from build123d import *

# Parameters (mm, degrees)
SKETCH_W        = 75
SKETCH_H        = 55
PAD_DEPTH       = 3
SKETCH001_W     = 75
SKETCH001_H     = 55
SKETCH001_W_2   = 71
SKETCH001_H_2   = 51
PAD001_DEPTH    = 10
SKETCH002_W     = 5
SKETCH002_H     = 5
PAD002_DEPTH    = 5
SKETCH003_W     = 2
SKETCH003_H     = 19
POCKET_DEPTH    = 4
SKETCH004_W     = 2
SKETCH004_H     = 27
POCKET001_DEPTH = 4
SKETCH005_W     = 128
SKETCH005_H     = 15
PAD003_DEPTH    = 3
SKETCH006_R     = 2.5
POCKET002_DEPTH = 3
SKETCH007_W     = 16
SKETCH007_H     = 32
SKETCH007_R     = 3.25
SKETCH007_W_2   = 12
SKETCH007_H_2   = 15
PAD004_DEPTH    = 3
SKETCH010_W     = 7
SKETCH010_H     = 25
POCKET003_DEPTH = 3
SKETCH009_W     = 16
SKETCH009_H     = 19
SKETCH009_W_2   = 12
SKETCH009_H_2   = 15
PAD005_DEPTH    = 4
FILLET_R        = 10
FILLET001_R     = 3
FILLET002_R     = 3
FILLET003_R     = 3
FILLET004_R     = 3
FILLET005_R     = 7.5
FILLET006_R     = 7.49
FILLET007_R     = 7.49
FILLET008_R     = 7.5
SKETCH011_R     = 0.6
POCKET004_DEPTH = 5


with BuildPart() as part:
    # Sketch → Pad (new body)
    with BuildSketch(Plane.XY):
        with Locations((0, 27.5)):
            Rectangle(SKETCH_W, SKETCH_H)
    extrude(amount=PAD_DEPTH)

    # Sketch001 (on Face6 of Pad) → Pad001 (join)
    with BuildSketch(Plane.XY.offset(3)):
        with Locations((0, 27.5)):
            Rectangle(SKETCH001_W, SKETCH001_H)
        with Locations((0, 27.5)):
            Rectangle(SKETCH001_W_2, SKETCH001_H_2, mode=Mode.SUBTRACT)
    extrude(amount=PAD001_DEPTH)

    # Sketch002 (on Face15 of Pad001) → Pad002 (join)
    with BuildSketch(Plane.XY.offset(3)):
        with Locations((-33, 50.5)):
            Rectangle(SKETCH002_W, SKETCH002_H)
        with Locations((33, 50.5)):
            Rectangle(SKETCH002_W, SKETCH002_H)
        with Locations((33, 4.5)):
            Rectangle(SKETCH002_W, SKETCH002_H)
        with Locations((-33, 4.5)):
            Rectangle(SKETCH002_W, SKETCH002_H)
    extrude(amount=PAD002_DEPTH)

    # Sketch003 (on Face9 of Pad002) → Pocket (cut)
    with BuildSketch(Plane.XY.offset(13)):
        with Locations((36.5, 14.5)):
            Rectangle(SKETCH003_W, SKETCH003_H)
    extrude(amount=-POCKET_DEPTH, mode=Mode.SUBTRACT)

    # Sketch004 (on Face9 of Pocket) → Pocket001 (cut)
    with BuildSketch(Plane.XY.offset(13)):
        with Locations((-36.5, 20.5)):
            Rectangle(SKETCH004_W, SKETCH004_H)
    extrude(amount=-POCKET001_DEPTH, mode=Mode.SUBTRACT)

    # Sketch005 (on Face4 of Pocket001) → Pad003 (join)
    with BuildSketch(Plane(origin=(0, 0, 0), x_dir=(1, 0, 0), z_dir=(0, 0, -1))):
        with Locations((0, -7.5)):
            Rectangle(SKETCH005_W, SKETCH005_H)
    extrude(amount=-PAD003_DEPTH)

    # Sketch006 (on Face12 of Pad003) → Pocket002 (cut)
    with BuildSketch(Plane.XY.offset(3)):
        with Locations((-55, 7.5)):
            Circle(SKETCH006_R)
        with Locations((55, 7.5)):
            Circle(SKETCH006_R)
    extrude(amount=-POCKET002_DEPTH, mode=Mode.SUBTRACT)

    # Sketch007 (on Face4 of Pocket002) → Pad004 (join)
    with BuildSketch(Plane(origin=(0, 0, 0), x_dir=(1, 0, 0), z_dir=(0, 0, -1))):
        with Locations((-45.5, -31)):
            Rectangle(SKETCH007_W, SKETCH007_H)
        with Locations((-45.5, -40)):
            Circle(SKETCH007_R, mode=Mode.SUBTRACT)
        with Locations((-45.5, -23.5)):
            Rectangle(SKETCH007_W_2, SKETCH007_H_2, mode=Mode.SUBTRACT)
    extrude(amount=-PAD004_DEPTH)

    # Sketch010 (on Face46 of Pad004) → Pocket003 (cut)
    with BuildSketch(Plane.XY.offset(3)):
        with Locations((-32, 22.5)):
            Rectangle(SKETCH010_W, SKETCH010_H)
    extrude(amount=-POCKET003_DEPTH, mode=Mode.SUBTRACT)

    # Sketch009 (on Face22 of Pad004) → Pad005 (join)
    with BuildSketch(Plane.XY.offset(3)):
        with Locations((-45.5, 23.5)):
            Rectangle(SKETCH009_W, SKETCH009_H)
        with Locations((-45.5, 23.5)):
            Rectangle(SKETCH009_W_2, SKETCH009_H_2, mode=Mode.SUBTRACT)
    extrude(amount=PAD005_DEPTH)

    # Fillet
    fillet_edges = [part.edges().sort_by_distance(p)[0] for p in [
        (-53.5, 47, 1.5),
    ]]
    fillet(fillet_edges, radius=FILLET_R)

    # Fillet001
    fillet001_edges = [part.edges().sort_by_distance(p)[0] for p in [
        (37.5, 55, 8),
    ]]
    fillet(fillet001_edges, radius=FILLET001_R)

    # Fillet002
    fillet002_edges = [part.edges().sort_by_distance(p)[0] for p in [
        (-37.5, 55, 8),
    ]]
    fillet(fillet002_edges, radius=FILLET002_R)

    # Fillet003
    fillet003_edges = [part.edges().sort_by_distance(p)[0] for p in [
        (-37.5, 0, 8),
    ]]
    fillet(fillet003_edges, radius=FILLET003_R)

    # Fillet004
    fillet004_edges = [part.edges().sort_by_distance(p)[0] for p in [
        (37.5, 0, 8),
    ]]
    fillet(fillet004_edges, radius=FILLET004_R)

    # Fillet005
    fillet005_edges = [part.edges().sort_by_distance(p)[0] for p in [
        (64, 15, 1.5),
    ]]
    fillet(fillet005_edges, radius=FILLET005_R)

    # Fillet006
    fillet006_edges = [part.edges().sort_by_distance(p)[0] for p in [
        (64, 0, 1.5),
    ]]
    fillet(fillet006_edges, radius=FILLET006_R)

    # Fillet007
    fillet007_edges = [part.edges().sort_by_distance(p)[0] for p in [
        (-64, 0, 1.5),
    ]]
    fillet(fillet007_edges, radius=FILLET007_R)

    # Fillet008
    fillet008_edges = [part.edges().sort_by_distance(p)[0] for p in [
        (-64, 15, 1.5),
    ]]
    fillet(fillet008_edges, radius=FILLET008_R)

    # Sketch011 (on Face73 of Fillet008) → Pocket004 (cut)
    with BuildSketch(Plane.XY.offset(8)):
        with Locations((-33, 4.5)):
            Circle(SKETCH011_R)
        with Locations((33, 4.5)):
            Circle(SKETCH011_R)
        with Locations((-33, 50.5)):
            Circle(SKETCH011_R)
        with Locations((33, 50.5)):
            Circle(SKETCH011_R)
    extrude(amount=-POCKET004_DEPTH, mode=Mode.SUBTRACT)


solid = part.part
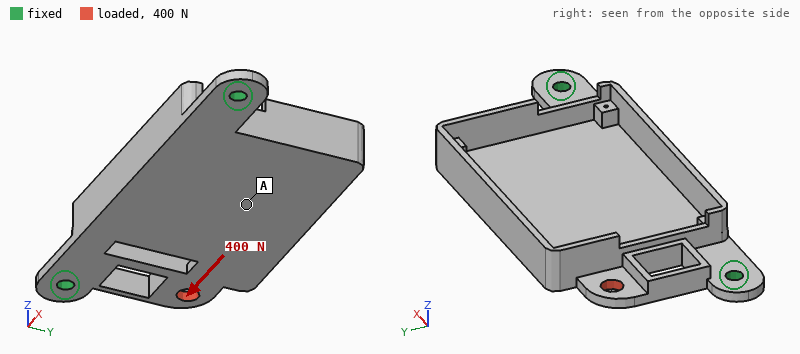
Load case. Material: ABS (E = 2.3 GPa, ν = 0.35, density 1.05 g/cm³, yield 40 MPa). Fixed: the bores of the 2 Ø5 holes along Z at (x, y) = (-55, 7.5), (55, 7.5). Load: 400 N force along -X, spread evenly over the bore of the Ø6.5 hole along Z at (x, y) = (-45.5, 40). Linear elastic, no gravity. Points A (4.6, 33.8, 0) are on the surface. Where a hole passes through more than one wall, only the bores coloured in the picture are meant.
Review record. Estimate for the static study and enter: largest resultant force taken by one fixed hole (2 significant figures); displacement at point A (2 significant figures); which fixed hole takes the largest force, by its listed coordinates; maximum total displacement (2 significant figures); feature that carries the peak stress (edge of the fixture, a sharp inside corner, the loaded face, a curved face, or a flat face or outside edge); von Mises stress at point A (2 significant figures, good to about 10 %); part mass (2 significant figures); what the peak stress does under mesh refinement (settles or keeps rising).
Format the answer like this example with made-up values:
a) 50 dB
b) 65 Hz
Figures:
a) 270 N
b) 0.23 mm
c) (55, 7.5)
d) 0.45 mm
e) edge of the fixture
f) 3.2 MPa
g) 21 g
h) keeps rising
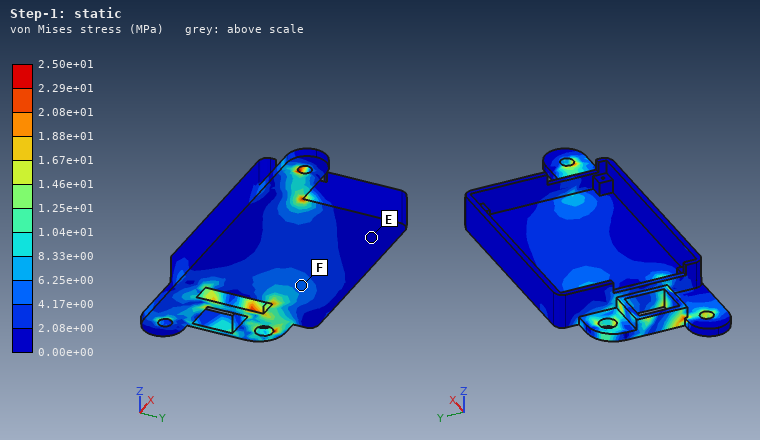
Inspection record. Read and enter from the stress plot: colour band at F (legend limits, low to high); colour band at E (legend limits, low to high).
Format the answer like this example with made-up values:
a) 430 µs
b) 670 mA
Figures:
a) 4.17e+00 to 6.25e+00 MPa
b) 0.00e+00 to 2.08e+00 MPa
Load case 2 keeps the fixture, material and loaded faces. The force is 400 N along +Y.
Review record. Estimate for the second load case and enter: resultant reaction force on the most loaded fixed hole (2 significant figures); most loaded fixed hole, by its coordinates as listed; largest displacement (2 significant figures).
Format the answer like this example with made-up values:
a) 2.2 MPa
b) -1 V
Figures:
a) 380 N
b) (-55, 7.5)
c) 0.84 mm
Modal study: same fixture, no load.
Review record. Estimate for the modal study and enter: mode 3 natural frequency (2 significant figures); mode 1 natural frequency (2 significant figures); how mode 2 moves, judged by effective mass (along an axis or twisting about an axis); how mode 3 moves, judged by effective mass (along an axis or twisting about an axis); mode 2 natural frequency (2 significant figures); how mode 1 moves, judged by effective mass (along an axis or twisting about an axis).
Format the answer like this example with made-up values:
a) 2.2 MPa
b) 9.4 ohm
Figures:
a) 690 Hz
b) 160 Hz
c) twisting about Y
d) along Z
e) 440 Hz
f) along Z
